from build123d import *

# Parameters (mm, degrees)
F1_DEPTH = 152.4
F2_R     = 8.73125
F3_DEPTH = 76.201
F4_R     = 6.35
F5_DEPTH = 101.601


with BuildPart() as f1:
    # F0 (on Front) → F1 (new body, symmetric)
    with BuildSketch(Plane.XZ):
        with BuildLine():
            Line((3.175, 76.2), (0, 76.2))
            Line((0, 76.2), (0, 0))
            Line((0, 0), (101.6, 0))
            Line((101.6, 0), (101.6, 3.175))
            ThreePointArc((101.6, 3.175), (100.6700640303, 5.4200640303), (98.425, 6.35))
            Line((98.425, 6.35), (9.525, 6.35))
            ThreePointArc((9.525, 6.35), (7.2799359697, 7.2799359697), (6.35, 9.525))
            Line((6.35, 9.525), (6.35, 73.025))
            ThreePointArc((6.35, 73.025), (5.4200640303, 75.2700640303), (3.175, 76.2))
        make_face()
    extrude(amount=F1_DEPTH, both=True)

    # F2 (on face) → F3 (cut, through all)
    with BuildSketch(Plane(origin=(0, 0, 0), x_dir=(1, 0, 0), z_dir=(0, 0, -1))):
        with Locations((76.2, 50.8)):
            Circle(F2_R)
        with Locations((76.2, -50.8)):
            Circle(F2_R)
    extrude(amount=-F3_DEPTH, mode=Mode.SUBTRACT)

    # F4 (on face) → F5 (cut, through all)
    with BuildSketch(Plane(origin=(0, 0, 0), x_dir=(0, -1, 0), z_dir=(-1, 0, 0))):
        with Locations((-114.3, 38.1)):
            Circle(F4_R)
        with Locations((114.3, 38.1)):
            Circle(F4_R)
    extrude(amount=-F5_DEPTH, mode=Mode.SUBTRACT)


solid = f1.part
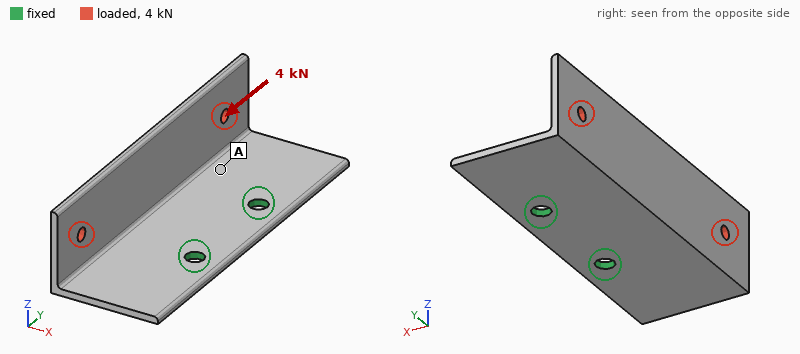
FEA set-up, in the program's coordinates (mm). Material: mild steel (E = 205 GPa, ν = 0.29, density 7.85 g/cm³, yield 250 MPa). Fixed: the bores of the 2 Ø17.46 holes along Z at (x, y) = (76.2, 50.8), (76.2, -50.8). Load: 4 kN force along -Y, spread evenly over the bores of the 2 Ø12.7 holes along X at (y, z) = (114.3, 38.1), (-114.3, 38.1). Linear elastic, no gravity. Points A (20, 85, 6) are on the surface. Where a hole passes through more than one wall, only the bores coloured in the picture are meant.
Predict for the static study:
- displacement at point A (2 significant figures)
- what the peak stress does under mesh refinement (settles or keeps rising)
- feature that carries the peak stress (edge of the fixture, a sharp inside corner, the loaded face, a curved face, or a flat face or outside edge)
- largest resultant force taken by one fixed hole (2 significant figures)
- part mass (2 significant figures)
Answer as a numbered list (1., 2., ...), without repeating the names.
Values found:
1. 0.14 mm
2. keeps rising
3. edge of the fixture
4. 3.3 kN
5. 2.6 kg
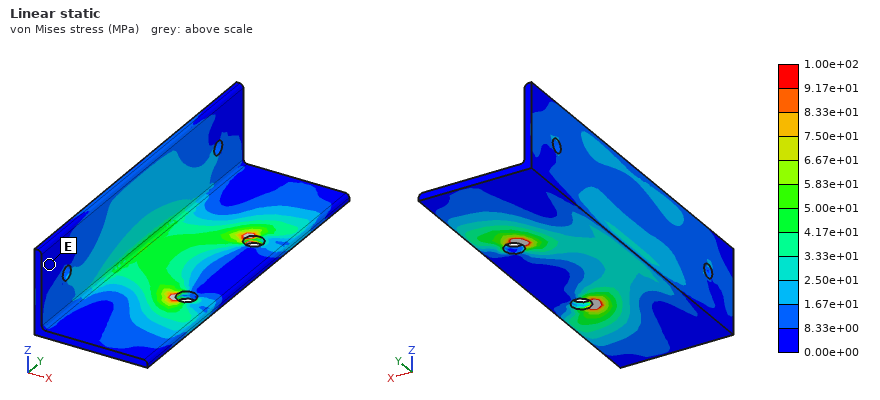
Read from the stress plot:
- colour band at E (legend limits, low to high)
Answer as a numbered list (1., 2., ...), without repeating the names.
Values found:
1. 0.00e+00 to 8.33e+00 MPa
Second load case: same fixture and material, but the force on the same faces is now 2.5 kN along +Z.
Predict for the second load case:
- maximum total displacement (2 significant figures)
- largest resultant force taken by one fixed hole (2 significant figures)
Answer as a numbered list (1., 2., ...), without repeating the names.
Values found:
1. 0.55 mm
2. 1.3 kN
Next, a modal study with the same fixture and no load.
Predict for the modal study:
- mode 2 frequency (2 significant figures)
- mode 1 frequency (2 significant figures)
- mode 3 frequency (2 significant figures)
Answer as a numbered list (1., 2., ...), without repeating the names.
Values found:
1. 330 Hz
2. 300 Hz
3. 730 Hz
